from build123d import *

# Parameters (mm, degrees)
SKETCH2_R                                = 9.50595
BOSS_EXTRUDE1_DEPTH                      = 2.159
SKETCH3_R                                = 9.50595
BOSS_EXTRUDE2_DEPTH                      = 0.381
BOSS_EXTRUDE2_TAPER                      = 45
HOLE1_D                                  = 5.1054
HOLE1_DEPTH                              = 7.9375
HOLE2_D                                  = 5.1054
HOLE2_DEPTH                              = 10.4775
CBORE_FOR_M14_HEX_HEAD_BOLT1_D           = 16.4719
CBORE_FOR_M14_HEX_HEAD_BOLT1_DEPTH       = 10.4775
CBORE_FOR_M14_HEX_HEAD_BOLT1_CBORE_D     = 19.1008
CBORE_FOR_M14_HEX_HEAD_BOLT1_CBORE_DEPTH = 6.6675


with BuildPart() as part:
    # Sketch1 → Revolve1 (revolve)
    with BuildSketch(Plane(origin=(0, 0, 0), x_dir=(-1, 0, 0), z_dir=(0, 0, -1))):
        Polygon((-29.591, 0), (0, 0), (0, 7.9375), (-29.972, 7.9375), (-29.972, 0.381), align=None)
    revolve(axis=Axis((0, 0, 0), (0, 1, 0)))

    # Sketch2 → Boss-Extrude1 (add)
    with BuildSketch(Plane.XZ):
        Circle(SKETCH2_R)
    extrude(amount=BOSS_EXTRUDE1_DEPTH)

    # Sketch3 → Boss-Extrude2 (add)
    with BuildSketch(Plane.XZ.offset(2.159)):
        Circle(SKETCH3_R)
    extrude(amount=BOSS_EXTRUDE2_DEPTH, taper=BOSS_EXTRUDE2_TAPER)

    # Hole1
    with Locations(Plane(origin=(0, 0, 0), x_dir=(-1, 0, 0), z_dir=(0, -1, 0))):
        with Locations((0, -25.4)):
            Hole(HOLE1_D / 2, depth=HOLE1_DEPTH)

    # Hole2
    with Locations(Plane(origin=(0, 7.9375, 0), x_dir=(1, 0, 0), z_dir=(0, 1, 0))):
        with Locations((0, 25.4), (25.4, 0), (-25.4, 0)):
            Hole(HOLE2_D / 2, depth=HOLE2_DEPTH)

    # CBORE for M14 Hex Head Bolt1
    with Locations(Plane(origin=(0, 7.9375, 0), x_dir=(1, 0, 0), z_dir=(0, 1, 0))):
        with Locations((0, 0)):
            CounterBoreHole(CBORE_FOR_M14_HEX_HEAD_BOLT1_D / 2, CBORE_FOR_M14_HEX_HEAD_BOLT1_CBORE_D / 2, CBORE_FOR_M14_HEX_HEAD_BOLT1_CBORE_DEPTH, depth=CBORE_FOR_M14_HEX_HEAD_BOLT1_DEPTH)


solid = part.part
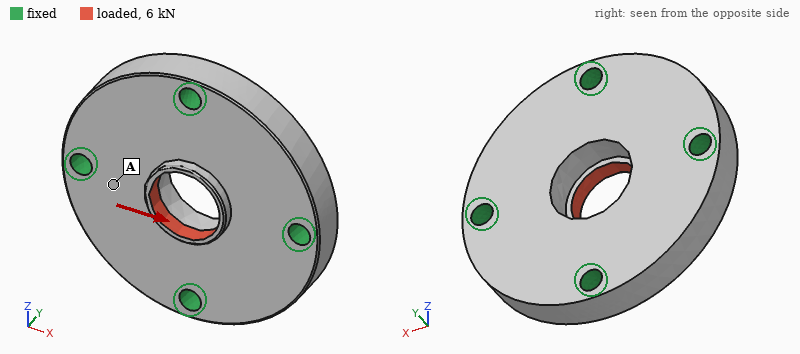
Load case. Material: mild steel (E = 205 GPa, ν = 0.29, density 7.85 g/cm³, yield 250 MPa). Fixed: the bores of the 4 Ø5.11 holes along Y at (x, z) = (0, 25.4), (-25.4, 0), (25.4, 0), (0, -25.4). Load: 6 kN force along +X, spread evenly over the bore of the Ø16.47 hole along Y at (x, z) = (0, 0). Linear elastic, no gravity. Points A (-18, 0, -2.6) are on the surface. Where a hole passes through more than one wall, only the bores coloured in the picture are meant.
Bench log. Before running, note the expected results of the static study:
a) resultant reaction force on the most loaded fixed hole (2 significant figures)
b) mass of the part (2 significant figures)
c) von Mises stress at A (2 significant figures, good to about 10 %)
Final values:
1.9 kN
150 g
27 MPa
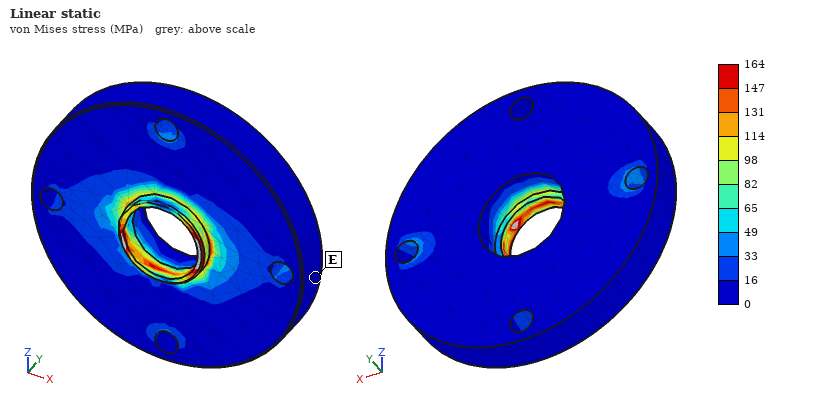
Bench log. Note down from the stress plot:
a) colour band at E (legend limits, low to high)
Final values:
0 to 16 MPa
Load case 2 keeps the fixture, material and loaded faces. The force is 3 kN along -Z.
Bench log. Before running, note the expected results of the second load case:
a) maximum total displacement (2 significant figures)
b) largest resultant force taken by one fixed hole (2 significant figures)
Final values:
5.5 µm
970 N
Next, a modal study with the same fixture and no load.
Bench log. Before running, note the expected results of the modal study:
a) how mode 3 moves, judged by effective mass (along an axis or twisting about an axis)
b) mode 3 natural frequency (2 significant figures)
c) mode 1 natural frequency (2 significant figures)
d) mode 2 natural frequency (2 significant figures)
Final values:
twisting about Z
24 kHz
22 kHz
22 kHz
